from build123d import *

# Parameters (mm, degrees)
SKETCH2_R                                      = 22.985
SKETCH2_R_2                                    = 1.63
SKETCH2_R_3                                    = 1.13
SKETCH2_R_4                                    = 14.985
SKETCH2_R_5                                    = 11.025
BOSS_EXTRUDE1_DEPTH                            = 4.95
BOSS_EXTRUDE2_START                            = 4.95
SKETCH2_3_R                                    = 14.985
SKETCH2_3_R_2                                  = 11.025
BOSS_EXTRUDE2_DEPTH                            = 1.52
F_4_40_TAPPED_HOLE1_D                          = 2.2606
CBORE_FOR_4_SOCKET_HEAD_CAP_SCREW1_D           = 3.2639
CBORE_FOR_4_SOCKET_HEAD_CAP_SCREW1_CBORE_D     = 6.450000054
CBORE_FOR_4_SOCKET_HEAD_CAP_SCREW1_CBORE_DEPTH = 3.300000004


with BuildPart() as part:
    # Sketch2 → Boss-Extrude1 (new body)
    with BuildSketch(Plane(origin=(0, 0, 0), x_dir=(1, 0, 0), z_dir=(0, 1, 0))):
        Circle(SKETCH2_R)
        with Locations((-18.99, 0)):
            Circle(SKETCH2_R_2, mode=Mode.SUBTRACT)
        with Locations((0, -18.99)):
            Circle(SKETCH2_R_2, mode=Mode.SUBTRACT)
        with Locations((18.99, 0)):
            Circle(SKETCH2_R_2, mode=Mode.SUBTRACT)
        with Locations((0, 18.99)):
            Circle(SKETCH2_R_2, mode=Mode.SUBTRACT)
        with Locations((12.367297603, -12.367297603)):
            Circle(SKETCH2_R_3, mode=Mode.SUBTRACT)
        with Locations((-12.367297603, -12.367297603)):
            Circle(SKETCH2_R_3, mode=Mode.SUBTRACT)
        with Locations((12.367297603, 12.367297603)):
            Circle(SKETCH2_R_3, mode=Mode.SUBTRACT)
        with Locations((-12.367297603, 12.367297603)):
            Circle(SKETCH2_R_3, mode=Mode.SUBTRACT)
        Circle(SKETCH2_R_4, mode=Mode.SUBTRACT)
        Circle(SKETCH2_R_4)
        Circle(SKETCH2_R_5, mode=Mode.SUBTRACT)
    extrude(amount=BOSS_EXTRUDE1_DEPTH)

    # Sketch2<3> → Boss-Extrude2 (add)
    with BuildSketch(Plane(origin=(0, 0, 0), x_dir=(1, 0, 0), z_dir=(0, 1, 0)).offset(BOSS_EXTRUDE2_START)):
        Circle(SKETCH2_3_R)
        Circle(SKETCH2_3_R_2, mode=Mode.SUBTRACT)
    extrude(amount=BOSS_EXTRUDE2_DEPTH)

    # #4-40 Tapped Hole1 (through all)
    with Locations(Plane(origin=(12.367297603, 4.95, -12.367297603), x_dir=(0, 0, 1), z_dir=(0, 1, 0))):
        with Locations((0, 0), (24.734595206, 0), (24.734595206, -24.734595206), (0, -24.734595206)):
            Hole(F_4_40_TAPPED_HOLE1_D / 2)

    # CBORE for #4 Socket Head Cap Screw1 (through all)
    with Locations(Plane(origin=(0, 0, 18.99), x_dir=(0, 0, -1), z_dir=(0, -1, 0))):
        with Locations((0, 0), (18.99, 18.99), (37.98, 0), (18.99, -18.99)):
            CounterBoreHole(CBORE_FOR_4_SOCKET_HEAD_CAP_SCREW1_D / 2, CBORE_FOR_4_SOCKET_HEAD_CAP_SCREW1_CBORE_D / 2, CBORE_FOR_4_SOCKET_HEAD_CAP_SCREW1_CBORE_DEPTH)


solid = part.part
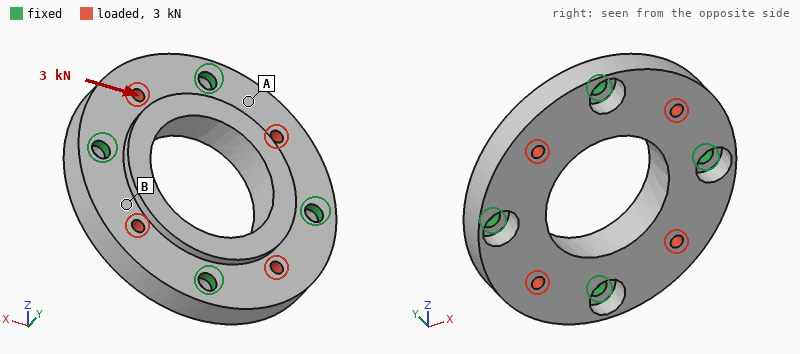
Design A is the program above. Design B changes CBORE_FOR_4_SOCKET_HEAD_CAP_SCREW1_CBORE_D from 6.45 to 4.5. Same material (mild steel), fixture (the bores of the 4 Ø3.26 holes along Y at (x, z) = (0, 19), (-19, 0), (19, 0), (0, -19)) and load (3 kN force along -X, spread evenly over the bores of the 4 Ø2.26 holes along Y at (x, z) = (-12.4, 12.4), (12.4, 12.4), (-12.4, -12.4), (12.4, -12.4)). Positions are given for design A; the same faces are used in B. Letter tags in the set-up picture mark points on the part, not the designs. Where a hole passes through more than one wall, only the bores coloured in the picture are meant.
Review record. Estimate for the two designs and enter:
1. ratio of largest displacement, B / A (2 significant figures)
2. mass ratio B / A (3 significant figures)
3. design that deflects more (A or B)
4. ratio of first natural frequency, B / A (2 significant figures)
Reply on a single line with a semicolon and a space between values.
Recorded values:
0.90; 1.04; A; 1.1
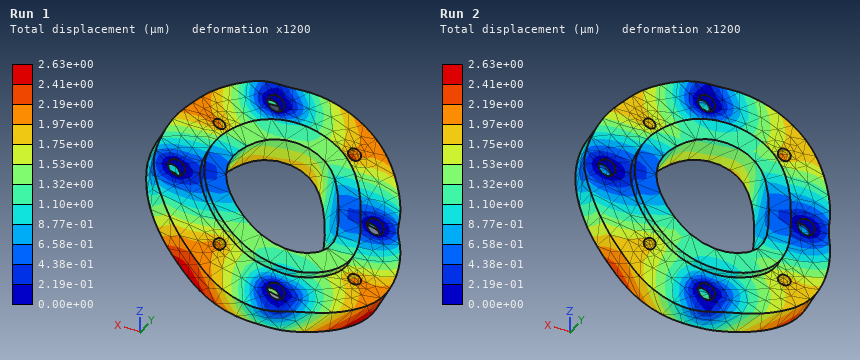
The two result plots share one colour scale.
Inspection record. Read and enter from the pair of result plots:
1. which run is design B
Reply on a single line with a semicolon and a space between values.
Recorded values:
Run 2
